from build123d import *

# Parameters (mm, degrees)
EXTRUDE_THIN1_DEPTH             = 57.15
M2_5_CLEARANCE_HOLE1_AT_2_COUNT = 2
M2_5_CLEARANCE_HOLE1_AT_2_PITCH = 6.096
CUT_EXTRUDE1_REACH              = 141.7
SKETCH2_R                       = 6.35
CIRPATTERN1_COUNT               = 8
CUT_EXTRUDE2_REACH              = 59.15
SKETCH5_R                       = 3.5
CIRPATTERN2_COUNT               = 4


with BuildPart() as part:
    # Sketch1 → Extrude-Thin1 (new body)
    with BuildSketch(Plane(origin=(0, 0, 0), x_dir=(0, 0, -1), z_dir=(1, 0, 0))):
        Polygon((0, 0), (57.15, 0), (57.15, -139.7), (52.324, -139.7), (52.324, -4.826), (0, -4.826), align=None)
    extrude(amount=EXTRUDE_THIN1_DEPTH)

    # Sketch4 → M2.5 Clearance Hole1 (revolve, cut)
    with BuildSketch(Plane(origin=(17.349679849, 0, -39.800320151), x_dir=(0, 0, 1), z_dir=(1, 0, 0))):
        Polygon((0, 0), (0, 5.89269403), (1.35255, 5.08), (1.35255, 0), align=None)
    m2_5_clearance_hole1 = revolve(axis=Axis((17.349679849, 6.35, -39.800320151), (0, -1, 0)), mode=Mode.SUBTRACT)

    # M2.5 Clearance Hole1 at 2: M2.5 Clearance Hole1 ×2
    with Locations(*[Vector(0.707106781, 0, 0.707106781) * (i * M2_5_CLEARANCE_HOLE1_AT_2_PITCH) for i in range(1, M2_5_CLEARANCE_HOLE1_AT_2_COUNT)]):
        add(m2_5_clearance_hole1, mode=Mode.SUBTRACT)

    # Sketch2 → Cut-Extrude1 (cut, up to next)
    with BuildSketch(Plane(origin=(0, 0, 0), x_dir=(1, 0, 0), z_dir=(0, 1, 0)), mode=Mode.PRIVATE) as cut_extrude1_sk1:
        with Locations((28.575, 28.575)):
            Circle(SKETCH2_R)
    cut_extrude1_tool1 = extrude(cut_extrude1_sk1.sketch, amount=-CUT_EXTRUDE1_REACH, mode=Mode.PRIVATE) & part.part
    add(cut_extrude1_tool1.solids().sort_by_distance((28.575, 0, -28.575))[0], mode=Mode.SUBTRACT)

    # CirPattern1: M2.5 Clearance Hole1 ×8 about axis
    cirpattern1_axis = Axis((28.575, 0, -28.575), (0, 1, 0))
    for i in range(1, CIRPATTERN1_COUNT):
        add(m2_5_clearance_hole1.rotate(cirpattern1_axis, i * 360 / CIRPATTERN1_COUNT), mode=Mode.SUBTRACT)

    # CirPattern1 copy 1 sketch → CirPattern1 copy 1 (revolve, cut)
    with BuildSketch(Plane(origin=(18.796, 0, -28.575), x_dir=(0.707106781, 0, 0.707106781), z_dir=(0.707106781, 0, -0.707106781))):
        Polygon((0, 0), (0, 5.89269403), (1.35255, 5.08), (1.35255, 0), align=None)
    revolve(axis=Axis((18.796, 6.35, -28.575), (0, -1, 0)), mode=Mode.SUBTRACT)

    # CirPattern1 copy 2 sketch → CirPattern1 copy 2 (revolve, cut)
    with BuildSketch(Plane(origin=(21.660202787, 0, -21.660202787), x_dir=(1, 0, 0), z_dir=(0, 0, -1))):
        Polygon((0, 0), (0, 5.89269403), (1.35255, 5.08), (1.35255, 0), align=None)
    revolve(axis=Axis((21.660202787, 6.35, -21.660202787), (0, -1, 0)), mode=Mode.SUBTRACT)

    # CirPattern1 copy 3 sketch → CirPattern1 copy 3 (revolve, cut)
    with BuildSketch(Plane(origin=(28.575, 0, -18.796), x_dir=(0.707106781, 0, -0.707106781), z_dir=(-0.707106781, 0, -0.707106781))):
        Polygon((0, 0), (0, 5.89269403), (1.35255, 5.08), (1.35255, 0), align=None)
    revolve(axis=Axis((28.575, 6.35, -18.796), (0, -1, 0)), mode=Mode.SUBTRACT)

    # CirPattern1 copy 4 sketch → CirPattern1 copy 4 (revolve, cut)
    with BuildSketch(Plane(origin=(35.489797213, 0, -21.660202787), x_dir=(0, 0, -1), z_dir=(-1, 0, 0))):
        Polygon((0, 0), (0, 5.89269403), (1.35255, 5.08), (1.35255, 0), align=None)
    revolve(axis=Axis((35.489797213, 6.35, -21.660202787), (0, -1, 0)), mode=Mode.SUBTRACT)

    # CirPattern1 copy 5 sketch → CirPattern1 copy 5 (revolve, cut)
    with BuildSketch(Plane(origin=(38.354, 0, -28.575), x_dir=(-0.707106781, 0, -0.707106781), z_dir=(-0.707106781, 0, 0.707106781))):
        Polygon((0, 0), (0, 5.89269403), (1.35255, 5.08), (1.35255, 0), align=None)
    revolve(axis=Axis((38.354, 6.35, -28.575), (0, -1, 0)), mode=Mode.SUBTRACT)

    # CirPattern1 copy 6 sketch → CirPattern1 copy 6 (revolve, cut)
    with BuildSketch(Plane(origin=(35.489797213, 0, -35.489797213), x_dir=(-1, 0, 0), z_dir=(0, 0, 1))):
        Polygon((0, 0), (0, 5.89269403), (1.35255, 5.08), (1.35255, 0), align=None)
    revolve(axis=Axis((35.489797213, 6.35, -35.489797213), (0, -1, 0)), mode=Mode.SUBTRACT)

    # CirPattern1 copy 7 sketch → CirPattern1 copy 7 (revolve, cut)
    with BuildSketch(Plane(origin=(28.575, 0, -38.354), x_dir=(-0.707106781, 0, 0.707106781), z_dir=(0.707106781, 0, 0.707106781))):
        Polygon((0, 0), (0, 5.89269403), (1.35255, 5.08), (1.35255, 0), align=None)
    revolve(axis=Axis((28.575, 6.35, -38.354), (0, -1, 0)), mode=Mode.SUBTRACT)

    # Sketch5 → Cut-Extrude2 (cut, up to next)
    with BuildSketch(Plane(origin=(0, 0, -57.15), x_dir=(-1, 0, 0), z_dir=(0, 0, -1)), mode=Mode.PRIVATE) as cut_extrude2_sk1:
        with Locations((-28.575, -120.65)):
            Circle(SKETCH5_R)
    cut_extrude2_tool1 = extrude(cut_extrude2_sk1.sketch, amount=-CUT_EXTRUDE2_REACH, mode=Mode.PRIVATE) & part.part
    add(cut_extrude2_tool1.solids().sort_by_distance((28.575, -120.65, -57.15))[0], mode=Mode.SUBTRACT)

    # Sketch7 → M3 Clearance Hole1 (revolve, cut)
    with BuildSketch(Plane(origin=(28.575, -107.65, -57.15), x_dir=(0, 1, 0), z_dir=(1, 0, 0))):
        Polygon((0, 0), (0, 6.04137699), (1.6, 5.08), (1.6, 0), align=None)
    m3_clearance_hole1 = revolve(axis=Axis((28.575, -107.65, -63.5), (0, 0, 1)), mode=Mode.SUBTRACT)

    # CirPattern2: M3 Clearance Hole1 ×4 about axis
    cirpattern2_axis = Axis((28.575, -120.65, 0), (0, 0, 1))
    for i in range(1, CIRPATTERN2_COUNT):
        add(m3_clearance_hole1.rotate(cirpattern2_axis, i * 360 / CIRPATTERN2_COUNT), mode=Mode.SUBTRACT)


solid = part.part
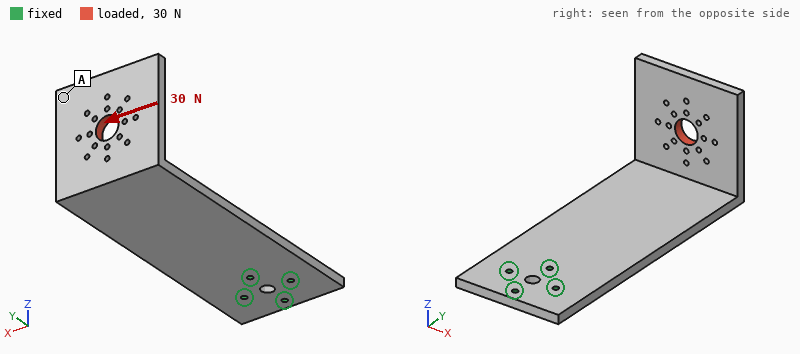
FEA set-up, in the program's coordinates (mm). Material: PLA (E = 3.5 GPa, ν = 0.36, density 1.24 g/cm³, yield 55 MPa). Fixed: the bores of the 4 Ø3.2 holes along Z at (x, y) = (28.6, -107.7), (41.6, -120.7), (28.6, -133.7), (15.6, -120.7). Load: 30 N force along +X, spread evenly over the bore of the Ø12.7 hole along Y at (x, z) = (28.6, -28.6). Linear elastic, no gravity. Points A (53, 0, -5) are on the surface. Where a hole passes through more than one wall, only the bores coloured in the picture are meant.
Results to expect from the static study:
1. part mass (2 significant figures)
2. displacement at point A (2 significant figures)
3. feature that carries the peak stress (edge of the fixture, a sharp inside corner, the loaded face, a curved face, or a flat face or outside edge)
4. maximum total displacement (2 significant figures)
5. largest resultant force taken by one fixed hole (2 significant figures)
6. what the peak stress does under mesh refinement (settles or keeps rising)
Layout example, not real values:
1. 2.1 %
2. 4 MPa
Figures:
1. 64 g
2. 1.7 mm
3. edge of the fixture
4. 1.9 mm
5. 79 N
6. keeps rising
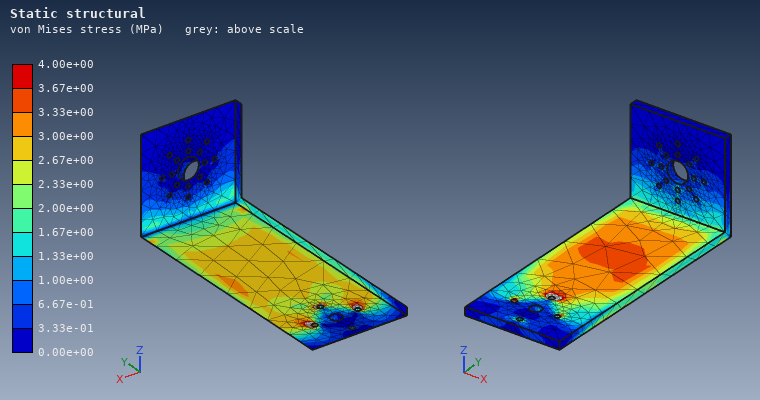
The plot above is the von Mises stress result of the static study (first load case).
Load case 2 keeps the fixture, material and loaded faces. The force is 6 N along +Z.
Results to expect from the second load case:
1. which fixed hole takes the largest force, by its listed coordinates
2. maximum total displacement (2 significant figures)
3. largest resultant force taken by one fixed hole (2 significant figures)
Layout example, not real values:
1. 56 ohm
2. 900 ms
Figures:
1. (28.6, -107.7)
2. 1.7 mm
3. 33 N
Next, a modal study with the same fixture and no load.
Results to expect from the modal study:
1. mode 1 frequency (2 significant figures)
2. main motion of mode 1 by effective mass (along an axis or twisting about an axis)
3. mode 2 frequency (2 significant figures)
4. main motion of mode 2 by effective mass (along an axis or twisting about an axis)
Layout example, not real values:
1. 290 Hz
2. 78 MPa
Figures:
1. 63 Hz
2. along Z
3. 160 Hz
4. along X
